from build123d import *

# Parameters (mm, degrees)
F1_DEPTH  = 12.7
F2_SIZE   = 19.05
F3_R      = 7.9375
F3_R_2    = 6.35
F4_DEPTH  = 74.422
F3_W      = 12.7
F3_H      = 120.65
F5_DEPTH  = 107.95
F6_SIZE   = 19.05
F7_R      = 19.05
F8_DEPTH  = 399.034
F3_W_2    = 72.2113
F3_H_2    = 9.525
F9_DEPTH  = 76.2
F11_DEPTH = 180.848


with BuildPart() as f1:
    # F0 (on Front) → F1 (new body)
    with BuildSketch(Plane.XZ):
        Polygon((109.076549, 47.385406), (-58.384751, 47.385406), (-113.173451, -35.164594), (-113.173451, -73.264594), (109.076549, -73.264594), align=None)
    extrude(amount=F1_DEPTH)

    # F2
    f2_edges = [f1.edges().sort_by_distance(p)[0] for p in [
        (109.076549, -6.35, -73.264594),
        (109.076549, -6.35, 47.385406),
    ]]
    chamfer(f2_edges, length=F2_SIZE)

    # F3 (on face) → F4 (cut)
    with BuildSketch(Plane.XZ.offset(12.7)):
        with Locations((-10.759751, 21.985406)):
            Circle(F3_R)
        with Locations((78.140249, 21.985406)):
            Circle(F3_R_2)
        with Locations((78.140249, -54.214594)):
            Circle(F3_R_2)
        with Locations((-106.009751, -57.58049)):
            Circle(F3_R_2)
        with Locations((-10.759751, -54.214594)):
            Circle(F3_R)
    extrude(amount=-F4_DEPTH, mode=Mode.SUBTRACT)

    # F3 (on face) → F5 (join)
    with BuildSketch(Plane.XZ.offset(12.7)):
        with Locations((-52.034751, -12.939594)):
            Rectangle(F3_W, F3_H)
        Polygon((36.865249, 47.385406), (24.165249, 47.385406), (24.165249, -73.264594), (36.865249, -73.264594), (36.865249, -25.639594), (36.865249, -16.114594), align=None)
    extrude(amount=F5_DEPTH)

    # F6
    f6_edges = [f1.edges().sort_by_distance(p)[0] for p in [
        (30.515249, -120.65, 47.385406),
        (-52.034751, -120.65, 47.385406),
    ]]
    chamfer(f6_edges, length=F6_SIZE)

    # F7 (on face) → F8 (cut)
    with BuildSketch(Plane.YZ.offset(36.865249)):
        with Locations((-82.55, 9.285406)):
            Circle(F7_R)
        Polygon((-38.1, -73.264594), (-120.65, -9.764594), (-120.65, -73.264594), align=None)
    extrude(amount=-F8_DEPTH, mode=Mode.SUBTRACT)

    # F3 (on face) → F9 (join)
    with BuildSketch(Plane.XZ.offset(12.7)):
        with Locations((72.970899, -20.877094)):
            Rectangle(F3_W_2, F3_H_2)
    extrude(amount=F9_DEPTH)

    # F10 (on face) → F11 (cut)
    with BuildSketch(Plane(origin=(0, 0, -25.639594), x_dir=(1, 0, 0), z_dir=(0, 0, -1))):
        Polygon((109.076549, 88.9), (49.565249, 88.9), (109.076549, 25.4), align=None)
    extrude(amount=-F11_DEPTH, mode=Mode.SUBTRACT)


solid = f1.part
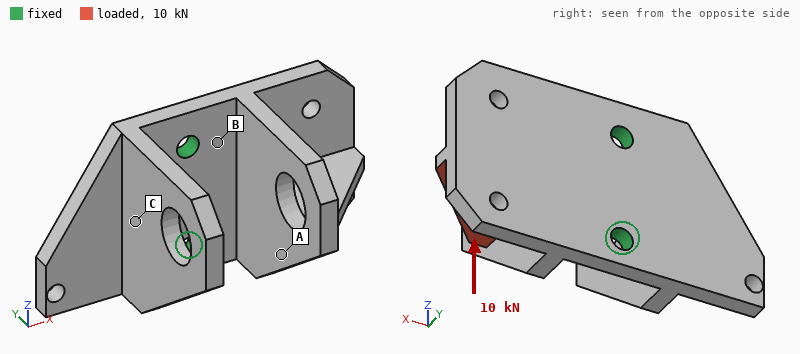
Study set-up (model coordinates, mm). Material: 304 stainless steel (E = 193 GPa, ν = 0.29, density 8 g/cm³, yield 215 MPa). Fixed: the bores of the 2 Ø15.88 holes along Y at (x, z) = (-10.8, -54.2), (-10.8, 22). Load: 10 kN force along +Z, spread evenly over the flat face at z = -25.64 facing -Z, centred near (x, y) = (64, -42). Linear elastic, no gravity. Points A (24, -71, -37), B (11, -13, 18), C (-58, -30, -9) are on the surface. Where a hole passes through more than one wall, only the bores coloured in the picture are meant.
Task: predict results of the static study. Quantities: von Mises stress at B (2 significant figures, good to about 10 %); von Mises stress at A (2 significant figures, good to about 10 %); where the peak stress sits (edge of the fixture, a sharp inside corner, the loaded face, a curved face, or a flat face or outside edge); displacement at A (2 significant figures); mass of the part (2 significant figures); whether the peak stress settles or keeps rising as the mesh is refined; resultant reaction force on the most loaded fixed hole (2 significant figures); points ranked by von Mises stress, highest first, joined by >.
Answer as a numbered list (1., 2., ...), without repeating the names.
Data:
1. 38 MPa
2. 18 MPa
3. edge of the fixture
4. 39 µm
5. 4.5 kg
6. keeps rising
7. 11 kN
8. B > A > C
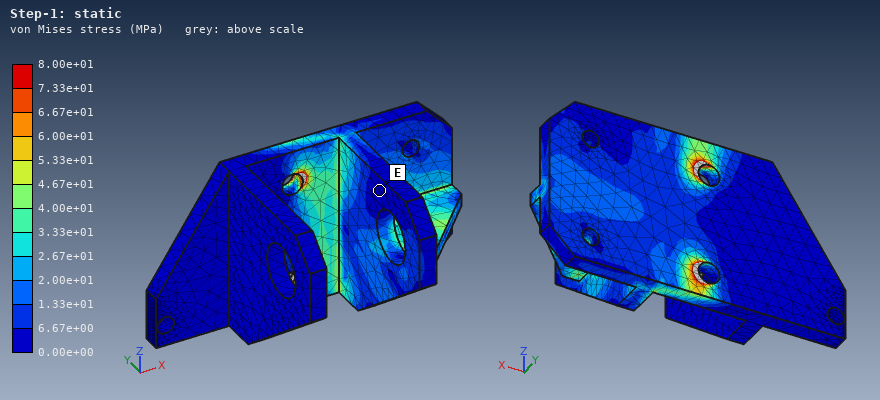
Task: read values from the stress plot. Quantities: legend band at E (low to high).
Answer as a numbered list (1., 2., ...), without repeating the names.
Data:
1. 0.00e+00 to 6.67e+00 MPa
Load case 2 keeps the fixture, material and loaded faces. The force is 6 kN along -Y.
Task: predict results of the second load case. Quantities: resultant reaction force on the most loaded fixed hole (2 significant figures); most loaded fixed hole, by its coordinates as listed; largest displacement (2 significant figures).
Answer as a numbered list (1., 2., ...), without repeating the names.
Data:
1. 3.7 kN
2. (-10.8, -54.2)
3. 0.39 mm
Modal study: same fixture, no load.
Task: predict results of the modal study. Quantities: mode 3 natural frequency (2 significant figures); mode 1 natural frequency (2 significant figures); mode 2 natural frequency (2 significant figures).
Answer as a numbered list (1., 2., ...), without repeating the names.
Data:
1. 1500 Hz
2. 540 Hz
3. 670 Hz
